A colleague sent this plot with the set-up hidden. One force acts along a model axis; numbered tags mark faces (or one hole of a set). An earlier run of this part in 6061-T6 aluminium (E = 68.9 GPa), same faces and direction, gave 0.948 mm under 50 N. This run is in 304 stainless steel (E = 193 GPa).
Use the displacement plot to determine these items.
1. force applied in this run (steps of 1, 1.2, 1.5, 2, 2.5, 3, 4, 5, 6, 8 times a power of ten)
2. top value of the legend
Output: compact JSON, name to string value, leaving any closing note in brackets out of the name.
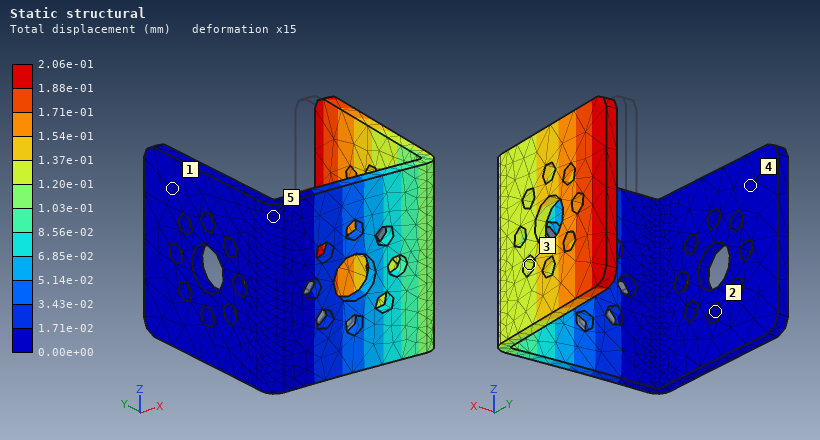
{"force applied in this run": "30 N", "top value of the legend": "2.06e-01 mm"}
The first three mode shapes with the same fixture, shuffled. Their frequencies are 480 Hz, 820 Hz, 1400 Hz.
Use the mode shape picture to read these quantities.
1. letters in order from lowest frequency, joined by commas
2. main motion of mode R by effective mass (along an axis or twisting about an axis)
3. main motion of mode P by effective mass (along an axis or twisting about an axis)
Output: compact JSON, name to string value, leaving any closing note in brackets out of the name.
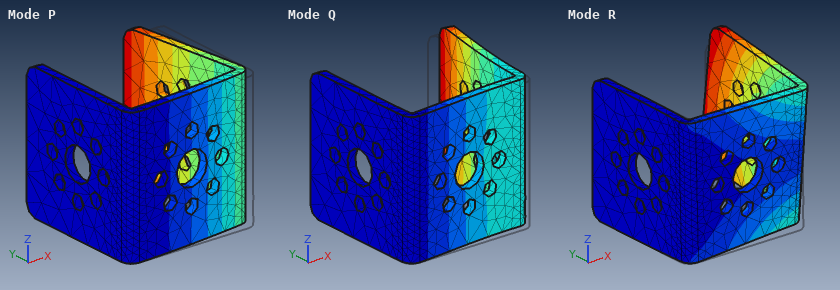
{"letters in order from lowest frequency, joined by commas": "P, R, Q", "main motion of mode R by effective mass": "along Z", "main motion of mode P by effective mass": "along Y"}
